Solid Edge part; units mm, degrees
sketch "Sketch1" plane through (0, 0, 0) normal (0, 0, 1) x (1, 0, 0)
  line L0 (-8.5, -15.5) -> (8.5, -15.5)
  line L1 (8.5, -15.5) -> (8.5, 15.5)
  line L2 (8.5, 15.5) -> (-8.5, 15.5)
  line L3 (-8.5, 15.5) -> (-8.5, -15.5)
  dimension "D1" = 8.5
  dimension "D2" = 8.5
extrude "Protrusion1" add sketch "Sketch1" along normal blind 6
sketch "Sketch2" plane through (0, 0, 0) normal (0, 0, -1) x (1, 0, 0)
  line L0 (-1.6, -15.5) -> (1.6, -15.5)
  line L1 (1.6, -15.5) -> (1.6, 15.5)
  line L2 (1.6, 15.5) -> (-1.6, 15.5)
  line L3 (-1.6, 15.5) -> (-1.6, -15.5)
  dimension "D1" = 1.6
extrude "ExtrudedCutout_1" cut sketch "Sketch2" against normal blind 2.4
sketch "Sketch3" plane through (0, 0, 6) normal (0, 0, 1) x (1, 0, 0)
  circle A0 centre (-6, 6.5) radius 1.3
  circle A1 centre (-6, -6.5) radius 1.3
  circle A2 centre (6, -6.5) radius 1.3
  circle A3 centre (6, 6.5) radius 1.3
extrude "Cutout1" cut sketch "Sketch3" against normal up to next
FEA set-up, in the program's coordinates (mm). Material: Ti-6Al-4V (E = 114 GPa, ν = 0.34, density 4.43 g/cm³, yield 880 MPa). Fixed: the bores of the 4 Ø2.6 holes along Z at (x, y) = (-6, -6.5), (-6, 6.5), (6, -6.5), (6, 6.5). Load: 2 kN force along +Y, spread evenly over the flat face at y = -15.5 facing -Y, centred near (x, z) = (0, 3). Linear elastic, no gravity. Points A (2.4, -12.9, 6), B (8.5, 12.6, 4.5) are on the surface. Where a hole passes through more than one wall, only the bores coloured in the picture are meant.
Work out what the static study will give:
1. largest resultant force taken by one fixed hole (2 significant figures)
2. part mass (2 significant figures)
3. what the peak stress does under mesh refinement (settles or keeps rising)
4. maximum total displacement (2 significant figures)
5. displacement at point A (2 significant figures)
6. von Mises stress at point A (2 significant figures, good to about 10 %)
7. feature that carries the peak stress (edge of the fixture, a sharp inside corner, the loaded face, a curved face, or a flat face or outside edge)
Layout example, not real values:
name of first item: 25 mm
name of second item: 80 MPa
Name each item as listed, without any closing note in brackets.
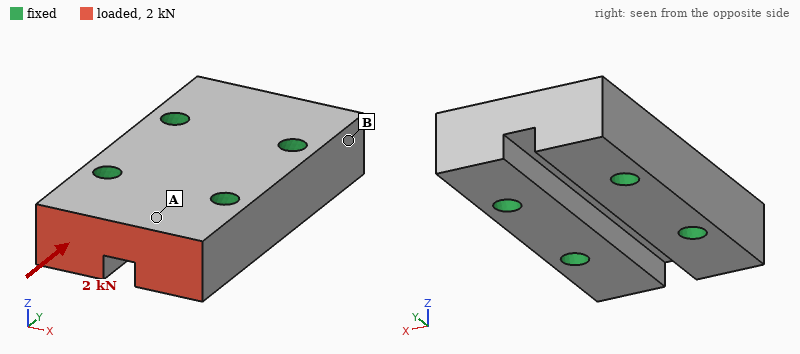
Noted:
largest resultant force taken by one fixed hole: 930 N
part mass: 12 g
what the peak stress does under mesh refinement: keeps rising
maximum total displacement: 2.0 µm
displacement at point A: 1.4 µm
von Mises stress at point A: 20 MPa
feature that carries the peak stress: edge of the fixture
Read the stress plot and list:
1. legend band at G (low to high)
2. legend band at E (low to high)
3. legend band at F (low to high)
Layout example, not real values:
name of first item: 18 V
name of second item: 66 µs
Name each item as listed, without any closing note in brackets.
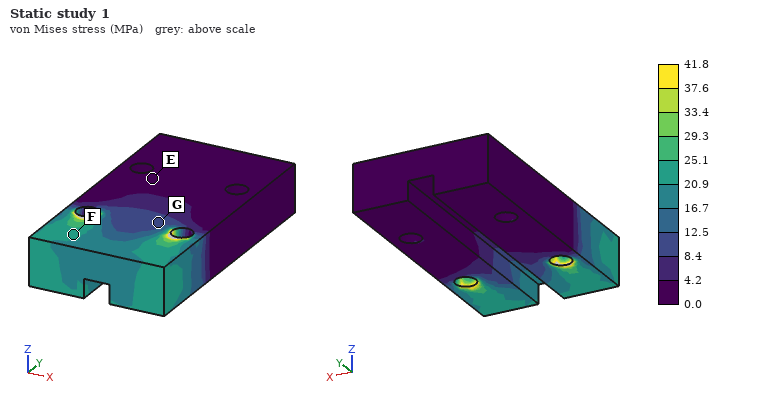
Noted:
legend band at G: 8.4 to 12.5 MPa
legend band at E: 0.0 to 4.2 MPa
legend band at F: 20.9 to 25.1 MPa
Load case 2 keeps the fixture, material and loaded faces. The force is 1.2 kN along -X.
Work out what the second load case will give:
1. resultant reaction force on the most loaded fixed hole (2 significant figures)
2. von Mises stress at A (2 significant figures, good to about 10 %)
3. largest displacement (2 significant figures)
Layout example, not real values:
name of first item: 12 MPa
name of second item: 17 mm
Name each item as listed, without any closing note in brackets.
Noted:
resultant reaction force on the most loaded fixed hole: 930 N
von Mises stress at A: 32 MPa
largest displacement: 6.2 µm
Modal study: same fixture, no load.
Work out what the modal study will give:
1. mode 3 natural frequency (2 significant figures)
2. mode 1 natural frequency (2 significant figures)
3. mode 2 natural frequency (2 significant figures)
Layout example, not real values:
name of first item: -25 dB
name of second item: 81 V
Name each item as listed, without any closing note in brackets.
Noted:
mode 3 natural frequency: 61 kHz
mode 1 natural frequency: 48 kHz
mode 2 natural frequency: 48 kHz
